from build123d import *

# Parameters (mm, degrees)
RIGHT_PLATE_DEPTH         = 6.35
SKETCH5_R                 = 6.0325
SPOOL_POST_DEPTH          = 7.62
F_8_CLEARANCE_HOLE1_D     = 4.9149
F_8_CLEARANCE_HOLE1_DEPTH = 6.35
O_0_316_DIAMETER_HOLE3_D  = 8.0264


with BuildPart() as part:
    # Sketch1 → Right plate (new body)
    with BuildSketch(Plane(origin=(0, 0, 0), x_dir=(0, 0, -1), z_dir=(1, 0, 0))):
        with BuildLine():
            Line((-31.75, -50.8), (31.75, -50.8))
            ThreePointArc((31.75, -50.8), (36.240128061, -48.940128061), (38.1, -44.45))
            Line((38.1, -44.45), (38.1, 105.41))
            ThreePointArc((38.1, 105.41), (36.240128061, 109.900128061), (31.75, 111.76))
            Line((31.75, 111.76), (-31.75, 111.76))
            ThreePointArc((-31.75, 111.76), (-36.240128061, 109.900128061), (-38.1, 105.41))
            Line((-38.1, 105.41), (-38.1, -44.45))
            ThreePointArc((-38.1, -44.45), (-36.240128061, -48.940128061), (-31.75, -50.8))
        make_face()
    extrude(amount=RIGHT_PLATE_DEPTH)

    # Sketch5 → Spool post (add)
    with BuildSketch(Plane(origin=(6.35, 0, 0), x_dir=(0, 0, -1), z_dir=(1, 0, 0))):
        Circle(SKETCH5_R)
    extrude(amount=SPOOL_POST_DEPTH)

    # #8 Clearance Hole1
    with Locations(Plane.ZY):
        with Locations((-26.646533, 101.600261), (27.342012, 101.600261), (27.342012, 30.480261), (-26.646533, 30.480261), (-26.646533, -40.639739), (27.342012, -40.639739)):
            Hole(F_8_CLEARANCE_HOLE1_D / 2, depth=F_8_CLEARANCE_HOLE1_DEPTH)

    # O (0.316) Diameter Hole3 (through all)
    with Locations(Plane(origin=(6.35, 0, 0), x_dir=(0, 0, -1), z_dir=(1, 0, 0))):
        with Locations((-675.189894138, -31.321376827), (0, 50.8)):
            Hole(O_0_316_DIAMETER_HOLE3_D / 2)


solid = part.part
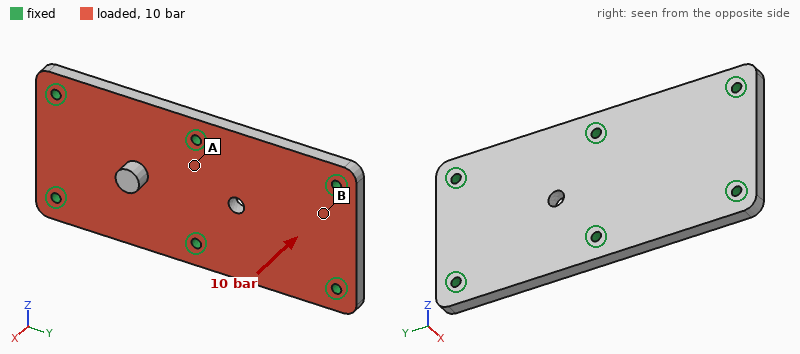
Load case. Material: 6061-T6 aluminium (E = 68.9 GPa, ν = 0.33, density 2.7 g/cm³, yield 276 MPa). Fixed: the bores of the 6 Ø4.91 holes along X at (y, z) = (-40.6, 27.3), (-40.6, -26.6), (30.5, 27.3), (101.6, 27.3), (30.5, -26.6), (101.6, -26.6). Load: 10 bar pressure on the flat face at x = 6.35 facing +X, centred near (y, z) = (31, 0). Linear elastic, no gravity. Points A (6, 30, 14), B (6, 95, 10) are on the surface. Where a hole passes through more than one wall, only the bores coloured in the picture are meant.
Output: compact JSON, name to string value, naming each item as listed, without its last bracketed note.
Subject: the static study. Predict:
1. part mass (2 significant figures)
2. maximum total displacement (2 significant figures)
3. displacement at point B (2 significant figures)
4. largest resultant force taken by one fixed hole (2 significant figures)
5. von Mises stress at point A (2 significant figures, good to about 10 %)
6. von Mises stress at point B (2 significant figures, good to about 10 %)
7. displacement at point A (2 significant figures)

{"part mass": "210 g", "maximum total displacement": "70 µm", "displacement at point B": "30 µm", "largest resultant force taken by one fixed hole": "2.8 kN", "von Mises stress at point A": "39 MPa", "von Mises stress at point B": "17 MPa", "displacement at point A": "23 µm"}
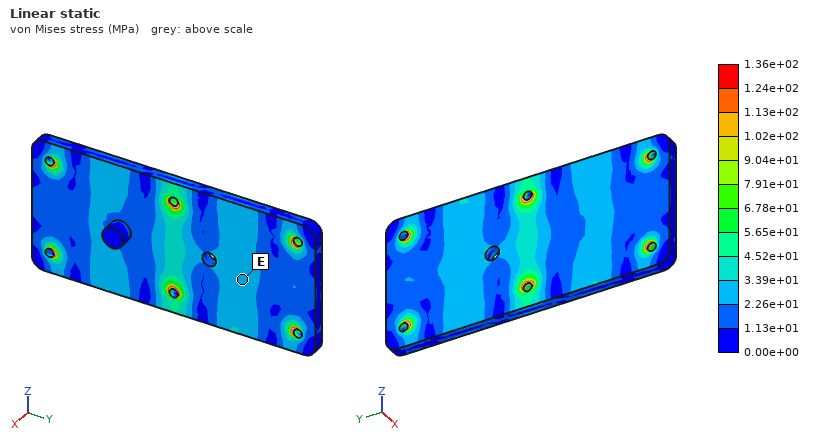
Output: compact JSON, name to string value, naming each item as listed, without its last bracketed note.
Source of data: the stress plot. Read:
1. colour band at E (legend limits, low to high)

{"colour band at E": "2.26e+01 to 3.39e+01 MPa"}
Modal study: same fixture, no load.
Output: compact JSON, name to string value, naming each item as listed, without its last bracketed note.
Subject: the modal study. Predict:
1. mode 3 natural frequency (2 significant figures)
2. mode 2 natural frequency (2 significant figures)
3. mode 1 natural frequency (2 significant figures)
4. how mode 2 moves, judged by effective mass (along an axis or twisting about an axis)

{"mode 3 natural frequency": "6900 Hz", "mode 2 natural frequency": "5400 Hz", "mode 1 natural frequency": "5000 Hz", "how mode 2 moves, judged by effective mass": "along X"}
